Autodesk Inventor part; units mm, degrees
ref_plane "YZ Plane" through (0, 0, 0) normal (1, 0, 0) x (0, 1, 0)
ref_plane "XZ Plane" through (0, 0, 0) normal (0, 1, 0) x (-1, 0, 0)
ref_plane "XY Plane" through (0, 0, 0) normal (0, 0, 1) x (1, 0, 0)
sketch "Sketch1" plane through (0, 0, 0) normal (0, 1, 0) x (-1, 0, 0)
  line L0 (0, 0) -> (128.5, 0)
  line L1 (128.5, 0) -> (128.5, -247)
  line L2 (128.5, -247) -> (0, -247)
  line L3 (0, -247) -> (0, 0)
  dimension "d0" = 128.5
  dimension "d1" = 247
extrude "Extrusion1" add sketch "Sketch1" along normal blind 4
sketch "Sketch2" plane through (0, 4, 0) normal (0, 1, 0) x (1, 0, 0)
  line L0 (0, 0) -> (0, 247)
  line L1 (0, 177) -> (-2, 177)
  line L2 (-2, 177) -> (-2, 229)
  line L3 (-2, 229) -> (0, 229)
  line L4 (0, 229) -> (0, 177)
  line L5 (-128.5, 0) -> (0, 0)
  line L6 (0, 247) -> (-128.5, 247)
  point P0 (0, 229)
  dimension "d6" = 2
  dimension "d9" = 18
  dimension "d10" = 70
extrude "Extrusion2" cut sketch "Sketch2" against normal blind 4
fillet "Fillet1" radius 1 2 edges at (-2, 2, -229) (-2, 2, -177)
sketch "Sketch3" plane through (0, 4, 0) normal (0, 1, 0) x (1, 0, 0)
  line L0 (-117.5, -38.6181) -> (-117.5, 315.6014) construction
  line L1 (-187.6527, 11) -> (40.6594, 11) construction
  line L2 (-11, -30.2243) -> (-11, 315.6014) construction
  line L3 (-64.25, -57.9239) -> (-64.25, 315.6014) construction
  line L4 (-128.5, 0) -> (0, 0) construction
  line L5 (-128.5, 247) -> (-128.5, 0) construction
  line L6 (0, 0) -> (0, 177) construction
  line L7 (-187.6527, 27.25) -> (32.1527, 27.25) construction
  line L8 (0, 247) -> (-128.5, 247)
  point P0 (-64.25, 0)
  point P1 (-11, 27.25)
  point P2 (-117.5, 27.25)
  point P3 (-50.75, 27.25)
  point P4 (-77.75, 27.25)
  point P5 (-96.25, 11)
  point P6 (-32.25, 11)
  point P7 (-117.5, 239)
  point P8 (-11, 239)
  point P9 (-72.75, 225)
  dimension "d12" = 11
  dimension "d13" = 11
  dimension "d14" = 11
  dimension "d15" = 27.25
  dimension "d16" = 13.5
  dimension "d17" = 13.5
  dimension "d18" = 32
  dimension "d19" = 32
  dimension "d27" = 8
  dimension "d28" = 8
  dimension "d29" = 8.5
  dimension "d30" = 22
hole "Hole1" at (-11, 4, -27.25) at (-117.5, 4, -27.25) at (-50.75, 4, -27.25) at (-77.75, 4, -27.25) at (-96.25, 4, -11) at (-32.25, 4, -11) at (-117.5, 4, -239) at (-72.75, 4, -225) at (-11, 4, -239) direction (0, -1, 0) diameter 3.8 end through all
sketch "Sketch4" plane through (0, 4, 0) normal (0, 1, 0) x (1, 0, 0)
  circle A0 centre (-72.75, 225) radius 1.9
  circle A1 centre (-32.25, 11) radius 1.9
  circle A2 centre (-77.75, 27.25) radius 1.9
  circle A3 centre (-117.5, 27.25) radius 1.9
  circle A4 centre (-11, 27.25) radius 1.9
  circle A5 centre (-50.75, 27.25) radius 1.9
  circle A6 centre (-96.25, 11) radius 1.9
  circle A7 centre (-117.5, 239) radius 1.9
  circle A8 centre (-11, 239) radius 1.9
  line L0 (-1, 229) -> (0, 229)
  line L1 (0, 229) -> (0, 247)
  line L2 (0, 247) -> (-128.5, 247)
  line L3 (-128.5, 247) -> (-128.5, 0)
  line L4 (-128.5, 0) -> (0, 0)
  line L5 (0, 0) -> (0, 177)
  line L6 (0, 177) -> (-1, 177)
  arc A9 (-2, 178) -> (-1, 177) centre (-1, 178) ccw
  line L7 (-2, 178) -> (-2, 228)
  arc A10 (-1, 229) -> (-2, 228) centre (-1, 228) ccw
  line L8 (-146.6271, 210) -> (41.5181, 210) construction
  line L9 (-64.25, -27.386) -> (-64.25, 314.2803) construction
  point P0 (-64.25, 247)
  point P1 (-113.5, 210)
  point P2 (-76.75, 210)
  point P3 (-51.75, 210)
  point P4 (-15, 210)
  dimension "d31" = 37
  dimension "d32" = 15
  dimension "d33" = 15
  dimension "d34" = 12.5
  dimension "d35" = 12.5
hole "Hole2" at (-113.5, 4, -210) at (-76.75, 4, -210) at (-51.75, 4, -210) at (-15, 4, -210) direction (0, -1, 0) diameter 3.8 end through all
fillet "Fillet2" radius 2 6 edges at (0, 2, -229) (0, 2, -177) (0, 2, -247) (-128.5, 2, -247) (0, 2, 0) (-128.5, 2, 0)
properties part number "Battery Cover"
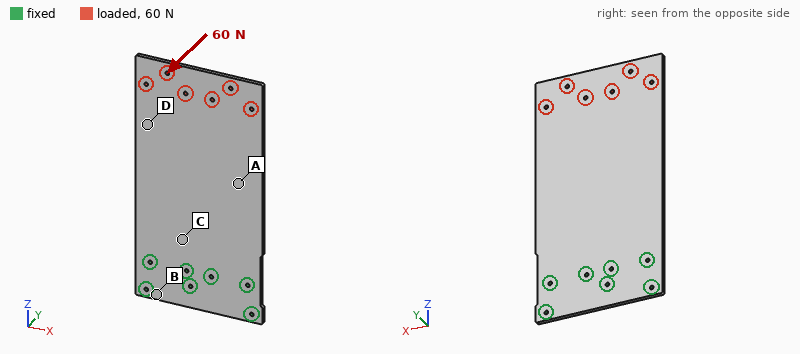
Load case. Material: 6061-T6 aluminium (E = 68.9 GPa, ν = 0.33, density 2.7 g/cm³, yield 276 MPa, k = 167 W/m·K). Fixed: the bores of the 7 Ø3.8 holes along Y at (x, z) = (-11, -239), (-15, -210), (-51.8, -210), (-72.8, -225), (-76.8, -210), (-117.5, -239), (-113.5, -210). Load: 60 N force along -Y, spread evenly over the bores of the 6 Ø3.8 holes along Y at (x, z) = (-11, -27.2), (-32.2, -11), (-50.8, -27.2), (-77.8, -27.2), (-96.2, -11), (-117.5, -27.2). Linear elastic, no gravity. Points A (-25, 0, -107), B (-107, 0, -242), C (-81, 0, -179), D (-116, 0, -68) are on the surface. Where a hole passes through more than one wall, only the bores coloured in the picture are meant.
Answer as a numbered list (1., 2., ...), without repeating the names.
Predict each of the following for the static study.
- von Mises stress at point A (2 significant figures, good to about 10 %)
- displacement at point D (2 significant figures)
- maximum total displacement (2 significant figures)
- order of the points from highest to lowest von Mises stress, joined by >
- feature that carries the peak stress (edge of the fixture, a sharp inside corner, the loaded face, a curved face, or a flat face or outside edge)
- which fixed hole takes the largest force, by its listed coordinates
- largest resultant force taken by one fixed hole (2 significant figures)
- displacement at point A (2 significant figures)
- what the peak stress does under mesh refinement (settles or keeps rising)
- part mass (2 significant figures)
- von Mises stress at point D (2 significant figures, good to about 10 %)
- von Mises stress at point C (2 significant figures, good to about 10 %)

1. 15 MPa
2. 1.7 mm
3. 3.3 mm
4. C > A > D > B
5. edge of the fixture
6. (-76.8, -210)
7. 130 N
8. 1.0 mm
9. keeps rising
10. 340 g
11. 8.3 MPa
12. 25 MPa
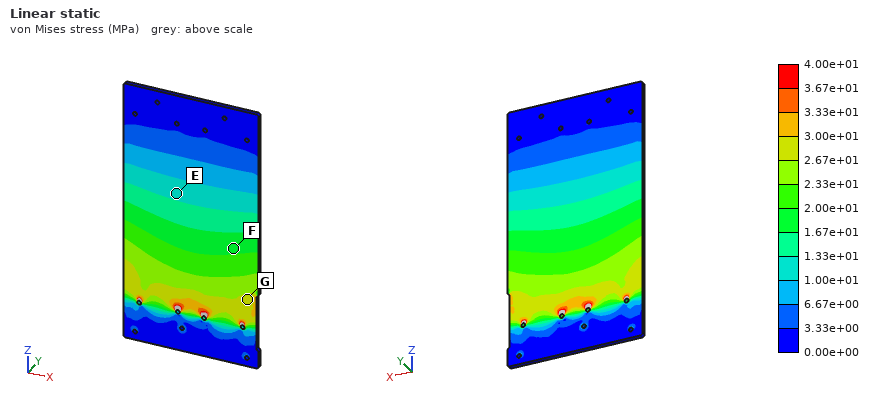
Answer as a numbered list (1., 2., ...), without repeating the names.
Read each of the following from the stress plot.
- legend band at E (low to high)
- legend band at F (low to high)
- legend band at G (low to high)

1. 1.00e+01 to 1.33e+01 MPa
2. 1.67e+01 to 2.00e+01 MPa
3. 2.67e+01 to 3.00e+01 MPa
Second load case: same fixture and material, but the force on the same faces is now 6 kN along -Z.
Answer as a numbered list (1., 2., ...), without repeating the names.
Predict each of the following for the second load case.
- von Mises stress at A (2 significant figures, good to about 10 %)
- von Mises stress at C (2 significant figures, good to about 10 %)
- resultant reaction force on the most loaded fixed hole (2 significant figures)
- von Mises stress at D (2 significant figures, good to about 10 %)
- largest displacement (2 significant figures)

1. 12 MPa
2. 12 MPa
3. 1.3 kN
4. 11 MPa
5. 37 µm
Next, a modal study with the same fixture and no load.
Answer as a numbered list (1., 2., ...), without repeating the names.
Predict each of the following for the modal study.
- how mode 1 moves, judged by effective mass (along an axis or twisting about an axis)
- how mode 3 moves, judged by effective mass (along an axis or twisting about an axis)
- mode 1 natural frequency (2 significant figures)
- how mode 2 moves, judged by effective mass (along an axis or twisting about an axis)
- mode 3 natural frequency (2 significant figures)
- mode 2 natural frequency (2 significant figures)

1. along Y
2. along Y
3. 75 Hz
4. twisting about Z
5. 470 Hz
6. 270 Hz
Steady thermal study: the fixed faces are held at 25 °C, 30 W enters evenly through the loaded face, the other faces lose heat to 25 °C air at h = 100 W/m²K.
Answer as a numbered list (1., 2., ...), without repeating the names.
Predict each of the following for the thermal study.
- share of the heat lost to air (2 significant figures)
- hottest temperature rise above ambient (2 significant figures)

1. 95 %
2. 16 K
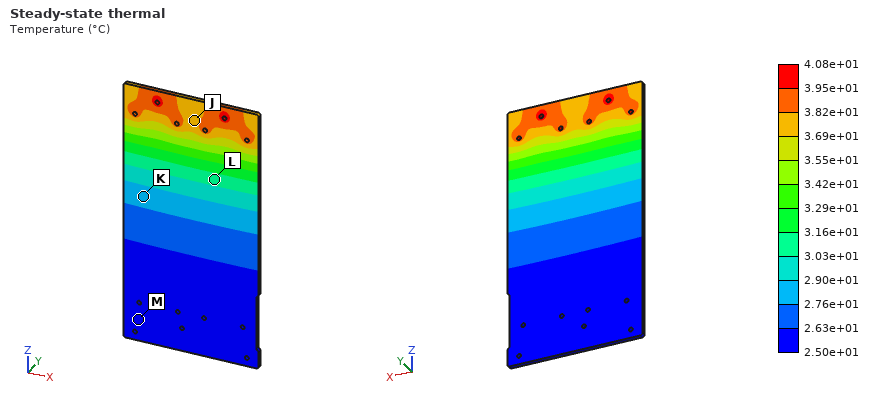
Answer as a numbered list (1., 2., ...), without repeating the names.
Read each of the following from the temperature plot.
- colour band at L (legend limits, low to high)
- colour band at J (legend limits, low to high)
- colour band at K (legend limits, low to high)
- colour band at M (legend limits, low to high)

1. 3.03e+01 to 3.16e+01 °C
2. 3.69e+01 to 3.82e+01 °C
3. 2.76e+01 to 2.90e+01 °C
4. 2.50e+01 to 2.63e+01 °C
